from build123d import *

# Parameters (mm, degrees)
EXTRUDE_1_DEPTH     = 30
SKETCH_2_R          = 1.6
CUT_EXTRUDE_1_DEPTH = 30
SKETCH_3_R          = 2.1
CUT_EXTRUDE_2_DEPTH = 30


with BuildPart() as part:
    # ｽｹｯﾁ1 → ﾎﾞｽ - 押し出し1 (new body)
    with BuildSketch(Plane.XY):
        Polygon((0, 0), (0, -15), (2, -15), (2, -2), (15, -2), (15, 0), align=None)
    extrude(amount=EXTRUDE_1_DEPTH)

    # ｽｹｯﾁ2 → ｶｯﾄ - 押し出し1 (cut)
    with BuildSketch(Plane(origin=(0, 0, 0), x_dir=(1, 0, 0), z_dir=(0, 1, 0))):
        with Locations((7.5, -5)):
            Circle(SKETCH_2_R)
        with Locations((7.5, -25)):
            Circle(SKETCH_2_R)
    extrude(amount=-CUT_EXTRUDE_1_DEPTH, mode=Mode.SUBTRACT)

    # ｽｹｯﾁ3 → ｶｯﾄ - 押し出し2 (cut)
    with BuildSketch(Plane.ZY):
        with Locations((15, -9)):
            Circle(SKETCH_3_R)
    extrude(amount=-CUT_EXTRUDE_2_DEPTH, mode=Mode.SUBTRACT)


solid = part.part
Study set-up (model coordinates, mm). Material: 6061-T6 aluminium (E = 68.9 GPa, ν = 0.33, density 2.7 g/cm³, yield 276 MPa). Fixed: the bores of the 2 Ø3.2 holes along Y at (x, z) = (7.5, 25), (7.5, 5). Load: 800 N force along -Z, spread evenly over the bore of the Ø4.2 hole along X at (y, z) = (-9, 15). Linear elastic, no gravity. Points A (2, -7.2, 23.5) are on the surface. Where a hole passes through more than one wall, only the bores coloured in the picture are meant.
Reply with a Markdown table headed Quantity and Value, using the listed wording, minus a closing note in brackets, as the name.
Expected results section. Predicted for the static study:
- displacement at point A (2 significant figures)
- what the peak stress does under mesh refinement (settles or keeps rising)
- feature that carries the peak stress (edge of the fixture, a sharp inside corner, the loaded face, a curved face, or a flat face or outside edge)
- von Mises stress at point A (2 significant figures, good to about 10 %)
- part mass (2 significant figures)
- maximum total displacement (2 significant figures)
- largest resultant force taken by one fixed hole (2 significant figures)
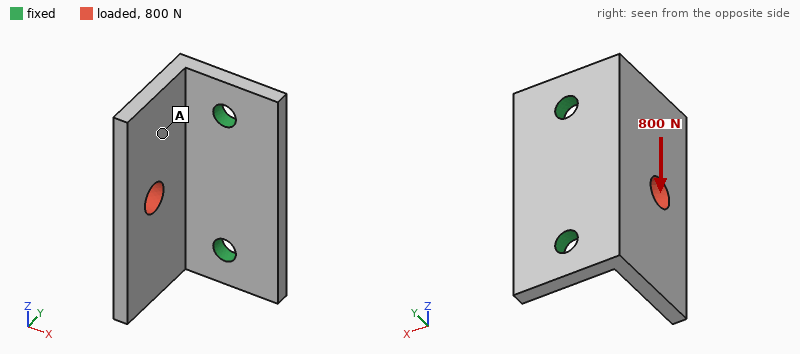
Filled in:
| Quantity | Value |
|---|---|
| displacement at point A | 36 µm |
| what the peak stress does under mesh refinement | keeps rising |
| feature that carries the peak stress | edge of the fixture |
| von Mises stress at point A | 44 MPa |
| part mass | 4.4 g |
| maximum total displacement | 81 µm |
| largest resultant force taken by one fixed hole | 550 N |
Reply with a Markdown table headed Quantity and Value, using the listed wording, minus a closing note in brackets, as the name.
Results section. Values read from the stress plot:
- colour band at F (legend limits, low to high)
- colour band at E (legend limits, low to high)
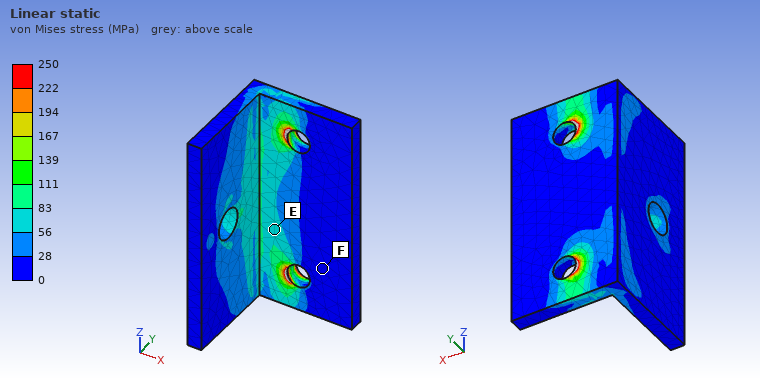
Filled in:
| Quantity | Value |
|---|---|
| colour band at F | 0 to 28 MPa |
| colour band at E | 56 to 83 MPa |
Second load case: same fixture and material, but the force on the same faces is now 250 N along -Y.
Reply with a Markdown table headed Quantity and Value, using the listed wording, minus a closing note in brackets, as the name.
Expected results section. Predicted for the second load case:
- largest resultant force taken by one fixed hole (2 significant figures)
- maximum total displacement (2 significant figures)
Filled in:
| Quantity | Value |
|---|---|
| largest resultant force taken by one fixed hole | 130 N |
| maximum total displacement | 53 µm |
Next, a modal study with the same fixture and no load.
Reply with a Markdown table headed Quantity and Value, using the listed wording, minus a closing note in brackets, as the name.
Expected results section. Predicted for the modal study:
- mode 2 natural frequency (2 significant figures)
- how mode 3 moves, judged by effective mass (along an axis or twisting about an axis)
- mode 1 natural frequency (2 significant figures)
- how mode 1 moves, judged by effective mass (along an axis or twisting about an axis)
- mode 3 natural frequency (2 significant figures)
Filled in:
| Quantity | Value |
|---|---|
| mode 2 natural frequency | 8800 Hz |
| how mode 3 moves, judged by effective mass | along Z |
| mode 1 natural frequency | 5100 Hz |
| how mode 1 moves, judged by effective mass | along X |
| mode 3 natural frequency | 16 kHz |
